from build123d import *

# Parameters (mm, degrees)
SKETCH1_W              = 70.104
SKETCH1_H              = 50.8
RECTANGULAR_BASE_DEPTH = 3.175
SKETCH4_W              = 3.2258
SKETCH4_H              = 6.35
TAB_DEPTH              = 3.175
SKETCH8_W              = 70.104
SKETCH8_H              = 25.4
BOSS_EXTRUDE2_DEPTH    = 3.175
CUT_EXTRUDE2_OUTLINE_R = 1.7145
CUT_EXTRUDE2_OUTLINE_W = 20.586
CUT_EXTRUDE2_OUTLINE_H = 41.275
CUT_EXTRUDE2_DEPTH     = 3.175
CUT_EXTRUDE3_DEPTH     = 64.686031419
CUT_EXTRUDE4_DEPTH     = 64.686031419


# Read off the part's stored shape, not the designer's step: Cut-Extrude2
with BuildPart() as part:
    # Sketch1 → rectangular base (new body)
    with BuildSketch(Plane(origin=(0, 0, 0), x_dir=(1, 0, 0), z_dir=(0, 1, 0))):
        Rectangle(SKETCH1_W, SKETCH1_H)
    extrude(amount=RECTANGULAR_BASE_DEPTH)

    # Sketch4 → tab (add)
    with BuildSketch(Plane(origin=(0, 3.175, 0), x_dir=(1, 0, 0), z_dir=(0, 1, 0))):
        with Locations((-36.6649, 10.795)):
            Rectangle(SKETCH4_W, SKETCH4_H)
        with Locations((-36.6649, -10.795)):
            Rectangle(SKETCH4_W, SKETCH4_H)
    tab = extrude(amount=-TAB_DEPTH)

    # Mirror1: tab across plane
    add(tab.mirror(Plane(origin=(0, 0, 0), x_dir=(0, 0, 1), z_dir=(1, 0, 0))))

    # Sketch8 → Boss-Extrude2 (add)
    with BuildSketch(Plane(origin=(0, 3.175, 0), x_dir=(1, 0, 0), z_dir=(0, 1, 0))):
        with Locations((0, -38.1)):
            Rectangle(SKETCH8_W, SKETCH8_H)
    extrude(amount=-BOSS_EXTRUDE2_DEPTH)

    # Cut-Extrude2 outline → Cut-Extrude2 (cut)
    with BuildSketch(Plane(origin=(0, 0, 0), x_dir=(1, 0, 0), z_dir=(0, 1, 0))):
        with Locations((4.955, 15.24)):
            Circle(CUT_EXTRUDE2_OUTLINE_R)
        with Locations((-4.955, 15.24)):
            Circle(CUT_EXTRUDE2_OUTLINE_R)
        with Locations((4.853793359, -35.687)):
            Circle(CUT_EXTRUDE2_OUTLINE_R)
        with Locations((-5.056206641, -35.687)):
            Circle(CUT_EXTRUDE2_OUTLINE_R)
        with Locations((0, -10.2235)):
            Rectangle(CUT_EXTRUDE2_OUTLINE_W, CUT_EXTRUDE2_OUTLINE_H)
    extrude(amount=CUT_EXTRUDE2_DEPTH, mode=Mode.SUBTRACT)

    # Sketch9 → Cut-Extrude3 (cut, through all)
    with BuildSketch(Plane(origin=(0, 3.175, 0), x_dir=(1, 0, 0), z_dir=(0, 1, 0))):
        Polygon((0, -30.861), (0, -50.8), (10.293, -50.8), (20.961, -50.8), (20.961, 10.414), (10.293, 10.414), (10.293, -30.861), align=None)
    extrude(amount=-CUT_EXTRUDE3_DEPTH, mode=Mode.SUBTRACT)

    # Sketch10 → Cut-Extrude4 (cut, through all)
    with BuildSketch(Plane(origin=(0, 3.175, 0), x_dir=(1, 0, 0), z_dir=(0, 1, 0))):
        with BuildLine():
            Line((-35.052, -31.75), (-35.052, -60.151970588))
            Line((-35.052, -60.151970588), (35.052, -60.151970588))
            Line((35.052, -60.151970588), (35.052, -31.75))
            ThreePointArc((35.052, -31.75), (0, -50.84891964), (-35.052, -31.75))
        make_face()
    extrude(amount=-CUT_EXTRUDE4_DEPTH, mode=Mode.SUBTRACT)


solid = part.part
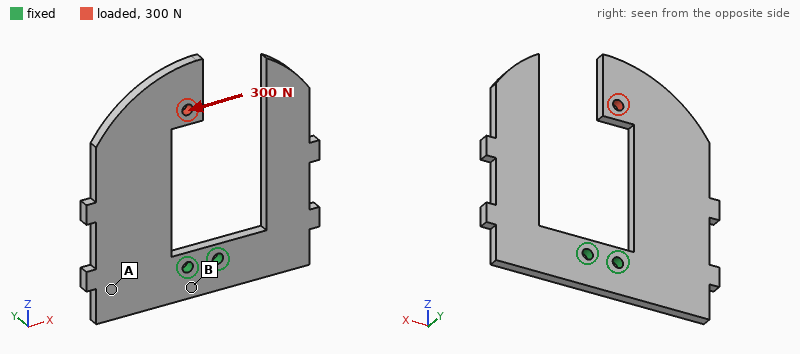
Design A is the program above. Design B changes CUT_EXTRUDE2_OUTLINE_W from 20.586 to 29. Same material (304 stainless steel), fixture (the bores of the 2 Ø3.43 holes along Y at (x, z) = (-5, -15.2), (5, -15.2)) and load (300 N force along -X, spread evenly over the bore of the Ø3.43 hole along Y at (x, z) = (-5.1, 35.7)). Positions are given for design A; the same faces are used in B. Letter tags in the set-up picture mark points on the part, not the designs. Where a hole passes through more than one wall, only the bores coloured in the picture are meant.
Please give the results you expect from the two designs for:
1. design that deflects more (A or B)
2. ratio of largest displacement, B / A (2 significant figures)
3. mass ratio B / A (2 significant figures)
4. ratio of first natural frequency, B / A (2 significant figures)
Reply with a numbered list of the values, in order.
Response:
1. B
2. 1.3
3. 0.95
4. 0.91
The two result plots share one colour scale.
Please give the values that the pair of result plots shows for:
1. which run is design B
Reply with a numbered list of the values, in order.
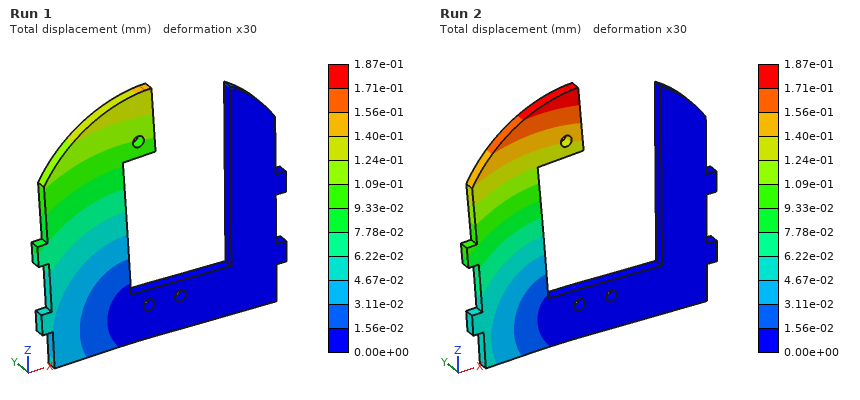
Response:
1. Run 2
